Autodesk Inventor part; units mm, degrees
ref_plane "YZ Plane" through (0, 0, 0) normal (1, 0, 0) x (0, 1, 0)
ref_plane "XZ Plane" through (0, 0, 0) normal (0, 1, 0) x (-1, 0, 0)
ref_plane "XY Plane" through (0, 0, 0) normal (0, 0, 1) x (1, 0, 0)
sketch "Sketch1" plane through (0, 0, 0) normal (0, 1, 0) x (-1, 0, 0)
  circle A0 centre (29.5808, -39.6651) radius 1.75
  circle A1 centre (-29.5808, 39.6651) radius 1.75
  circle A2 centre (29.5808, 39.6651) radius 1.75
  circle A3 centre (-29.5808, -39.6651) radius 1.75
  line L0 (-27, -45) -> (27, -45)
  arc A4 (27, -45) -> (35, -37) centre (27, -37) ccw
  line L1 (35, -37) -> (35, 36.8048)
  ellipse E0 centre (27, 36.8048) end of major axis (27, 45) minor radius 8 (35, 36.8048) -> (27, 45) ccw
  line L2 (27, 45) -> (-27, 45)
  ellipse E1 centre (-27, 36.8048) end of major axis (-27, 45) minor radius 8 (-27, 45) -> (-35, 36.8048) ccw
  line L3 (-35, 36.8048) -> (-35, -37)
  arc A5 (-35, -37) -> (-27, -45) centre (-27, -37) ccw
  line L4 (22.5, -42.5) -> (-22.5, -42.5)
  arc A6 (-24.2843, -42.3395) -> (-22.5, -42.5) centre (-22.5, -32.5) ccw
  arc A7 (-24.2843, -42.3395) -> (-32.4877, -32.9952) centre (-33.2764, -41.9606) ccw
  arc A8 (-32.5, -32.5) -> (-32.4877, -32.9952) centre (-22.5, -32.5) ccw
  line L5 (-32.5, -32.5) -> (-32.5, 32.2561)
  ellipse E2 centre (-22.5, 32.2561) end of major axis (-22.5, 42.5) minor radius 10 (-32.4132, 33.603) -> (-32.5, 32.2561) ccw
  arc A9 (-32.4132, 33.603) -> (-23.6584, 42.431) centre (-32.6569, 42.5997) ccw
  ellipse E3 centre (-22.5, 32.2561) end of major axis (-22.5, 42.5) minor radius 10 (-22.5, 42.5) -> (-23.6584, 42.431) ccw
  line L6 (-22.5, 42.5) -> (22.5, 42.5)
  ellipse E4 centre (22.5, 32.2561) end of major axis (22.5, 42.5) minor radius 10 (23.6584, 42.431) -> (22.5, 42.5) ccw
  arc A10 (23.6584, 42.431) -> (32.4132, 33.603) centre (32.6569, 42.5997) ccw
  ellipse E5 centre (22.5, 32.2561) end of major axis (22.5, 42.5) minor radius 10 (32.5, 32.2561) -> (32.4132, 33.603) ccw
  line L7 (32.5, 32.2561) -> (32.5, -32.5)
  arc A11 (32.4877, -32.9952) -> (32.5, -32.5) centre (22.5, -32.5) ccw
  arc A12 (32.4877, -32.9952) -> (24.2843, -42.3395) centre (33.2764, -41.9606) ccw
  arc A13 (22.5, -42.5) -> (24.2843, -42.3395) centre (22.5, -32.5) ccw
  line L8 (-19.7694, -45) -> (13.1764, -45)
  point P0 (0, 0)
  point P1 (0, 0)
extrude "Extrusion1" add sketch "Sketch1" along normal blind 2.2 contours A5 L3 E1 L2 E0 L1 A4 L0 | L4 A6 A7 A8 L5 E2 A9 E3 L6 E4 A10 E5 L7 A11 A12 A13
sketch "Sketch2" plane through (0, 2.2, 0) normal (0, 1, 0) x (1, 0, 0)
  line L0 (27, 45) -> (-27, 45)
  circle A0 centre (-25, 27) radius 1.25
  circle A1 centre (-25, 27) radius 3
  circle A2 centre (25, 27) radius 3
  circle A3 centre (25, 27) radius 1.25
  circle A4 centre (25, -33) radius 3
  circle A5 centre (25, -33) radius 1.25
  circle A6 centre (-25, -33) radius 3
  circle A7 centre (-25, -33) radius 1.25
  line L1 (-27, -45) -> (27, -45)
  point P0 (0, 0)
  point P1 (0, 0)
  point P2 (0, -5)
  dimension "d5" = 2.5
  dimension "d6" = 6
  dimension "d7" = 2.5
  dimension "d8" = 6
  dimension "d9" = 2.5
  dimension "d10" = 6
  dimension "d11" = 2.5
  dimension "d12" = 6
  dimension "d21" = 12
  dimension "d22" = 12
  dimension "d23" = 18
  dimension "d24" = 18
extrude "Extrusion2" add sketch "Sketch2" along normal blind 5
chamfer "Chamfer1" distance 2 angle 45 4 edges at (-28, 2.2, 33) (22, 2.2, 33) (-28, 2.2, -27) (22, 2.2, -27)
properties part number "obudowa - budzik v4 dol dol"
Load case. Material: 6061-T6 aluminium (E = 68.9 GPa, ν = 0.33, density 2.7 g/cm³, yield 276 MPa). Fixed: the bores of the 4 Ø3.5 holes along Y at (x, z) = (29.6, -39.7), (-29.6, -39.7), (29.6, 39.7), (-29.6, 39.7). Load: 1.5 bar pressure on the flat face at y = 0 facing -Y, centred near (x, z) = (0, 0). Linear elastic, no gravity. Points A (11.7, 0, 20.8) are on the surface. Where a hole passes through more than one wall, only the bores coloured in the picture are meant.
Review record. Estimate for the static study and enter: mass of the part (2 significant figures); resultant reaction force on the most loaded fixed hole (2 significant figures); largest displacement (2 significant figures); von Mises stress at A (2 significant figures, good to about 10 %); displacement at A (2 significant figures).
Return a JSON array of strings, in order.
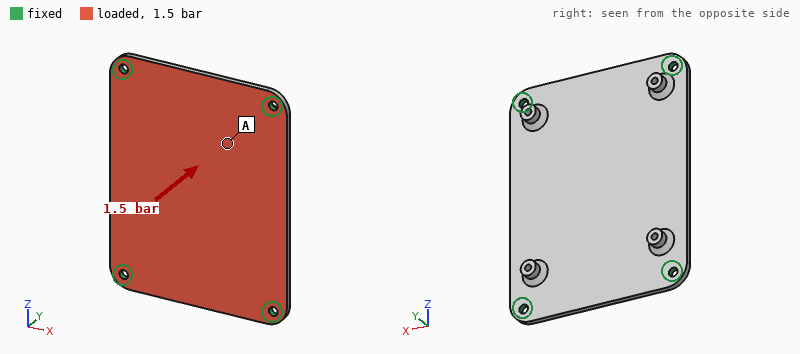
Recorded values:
["39 g", "240 N", "0.41 mm", "28 MPa", "0.27 mm"]
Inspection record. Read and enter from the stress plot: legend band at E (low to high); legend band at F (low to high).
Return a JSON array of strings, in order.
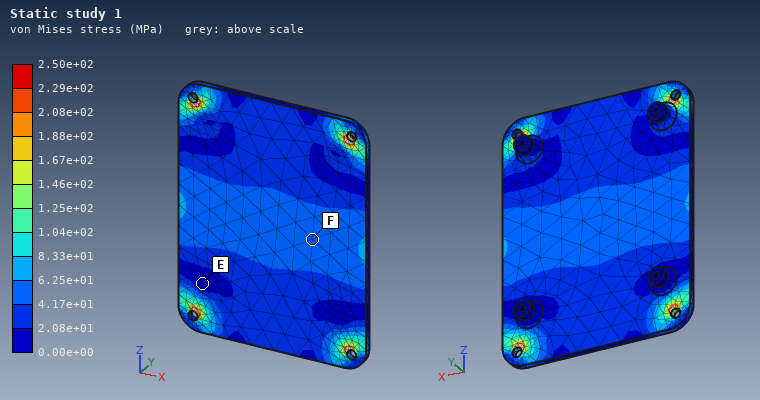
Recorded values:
["0.00e+00 to 2.08e+01 MPa", "4.17e+01 to 6.25e+01 MPa"]
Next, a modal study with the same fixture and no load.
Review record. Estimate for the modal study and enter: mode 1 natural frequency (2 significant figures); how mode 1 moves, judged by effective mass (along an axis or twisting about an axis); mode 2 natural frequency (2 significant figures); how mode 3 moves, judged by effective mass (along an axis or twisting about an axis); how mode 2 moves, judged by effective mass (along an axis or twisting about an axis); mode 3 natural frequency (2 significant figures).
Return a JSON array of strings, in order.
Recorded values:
["1500 Hz", "along Y", "2400 Hz", "twisting about X", "twisting about Z", "3200 Hz"]
